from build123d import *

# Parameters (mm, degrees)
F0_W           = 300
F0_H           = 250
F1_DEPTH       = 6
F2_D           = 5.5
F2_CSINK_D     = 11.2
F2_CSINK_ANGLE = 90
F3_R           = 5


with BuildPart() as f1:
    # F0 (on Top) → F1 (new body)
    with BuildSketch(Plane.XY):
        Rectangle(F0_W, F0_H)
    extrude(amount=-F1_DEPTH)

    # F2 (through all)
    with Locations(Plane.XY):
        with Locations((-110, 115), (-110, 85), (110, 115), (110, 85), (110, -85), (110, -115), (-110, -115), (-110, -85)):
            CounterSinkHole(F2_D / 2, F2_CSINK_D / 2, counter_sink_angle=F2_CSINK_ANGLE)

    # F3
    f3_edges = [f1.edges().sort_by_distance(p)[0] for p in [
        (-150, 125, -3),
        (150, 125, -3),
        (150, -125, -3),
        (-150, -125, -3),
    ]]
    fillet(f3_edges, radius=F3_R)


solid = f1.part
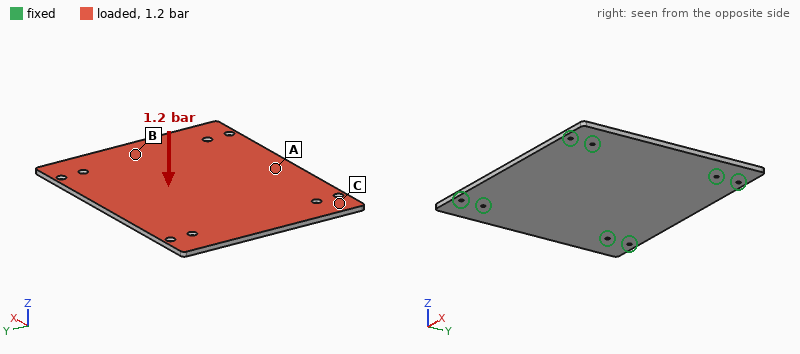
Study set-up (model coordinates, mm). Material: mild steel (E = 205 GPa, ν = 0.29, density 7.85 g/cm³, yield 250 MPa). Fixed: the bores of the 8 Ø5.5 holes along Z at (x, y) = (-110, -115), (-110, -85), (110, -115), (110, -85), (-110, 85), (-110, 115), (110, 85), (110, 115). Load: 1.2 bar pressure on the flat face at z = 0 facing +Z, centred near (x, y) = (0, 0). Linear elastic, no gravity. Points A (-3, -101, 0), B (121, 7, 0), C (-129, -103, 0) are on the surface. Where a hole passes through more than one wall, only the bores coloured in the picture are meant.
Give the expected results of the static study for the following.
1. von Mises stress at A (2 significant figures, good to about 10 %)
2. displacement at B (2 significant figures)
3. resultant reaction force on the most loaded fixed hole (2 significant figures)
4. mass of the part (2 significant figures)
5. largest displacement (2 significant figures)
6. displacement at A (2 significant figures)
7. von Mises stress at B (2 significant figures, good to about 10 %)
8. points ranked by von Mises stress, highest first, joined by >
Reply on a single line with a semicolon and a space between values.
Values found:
56 MPa; 0.11 mm; 3.2 kN; 3.5 kg; 0.41 mm; 0.31 mm; 37 MPa; A > B > C
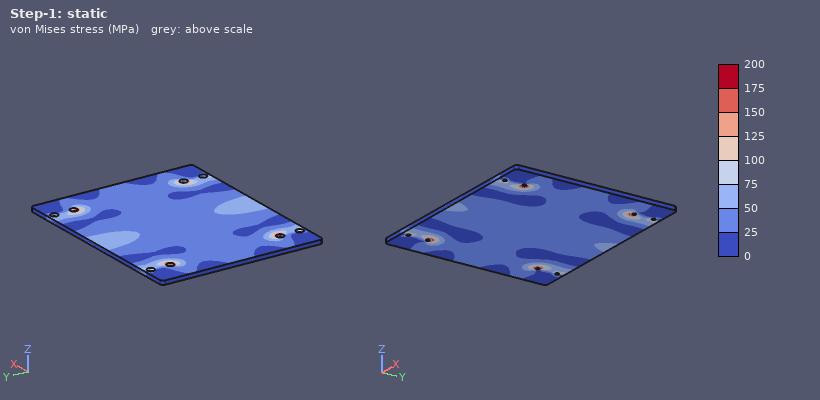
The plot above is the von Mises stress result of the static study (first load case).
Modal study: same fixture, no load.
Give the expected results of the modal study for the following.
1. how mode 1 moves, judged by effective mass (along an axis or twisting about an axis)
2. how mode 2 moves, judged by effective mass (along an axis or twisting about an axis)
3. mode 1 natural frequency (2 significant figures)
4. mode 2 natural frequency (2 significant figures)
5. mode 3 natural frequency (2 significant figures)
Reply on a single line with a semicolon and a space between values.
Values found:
along Z; twisting about X; 470 Hz; 690 Hz; 870 Hz
